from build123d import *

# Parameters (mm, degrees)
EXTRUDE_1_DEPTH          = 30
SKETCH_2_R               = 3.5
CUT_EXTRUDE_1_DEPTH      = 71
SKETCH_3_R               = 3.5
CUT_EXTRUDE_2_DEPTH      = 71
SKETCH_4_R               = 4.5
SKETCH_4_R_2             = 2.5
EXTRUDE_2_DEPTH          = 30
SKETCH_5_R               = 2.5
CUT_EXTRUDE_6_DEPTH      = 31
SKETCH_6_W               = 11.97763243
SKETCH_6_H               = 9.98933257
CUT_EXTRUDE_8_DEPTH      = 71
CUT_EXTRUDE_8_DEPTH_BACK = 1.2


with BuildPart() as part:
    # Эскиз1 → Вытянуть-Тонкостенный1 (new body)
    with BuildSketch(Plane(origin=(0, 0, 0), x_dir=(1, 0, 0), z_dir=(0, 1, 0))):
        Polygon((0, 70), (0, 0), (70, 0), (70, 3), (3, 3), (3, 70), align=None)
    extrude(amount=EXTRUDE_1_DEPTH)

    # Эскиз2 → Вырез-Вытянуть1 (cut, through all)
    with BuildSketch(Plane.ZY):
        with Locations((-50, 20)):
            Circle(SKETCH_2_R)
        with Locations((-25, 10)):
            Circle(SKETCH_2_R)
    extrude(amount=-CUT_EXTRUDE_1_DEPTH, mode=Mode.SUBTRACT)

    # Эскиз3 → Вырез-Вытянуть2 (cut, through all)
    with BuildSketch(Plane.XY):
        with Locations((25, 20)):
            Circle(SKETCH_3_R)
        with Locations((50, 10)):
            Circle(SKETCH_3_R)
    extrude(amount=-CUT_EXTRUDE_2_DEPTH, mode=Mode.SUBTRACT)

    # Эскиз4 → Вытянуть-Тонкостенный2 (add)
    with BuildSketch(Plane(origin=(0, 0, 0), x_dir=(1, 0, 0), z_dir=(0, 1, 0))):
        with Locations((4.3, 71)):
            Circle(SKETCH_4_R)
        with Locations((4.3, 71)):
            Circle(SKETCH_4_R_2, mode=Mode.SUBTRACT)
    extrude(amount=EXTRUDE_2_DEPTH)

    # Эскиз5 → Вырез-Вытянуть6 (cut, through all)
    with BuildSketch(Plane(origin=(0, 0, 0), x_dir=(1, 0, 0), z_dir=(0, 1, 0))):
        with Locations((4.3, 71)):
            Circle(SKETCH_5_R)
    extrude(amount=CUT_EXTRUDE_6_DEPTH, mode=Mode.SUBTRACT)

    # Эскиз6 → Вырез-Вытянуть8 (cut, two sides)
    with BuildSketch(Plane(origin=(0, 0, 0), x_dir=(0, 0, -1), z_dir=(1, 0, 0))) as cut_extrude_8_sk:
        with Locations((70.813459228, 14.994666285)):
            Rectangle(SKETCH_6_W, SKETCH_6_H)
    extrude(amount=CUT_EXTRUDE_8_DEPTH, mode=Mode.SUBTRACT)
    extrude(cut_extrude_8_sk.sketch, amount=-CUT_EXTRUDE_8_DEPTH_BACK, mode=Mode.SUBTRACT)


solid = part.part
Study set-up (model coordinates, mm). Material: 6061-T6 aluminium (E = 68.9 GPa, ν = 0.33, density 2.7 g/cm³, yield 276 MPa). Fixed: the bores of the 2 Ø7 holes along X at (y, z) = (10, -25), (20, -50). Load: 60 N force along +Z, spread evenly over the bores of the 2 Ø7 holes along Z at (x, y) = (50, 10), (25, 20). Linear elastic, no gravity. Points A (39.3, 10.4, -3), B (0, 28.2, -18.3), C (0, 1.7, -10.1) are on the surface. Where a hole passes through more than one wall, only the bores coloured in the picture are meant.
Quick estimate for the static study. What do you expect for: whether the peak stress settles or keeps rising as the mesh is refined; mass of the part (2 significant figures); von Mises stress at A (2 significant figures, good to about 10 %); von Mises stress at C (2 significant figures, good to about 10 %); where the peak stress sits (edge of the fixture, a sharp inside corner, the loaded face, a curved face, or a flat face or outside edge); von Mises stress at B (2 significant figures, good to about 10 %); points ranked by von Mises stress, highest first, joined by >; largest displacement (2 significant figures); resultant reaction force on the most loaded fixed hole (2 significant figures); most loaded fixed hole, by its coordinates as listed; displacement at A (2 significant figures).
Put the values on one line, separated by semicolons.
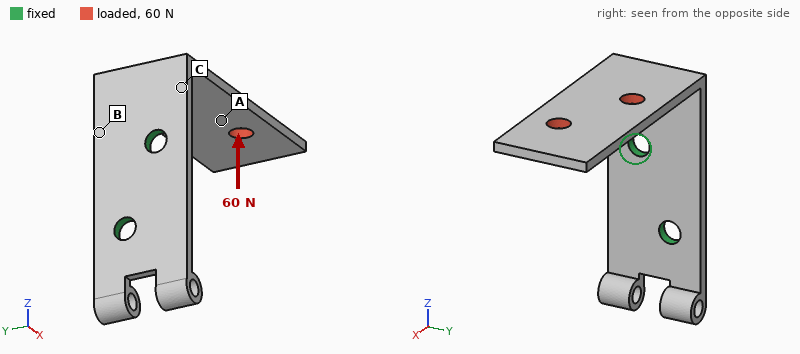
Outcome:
keeps rising; 34 g; 8.6 MPa; 51 MPa; edge of the fixture; 37 MPa; C > B > A; 1.2 mm; 51 N; (10, -25); 0.58 mm
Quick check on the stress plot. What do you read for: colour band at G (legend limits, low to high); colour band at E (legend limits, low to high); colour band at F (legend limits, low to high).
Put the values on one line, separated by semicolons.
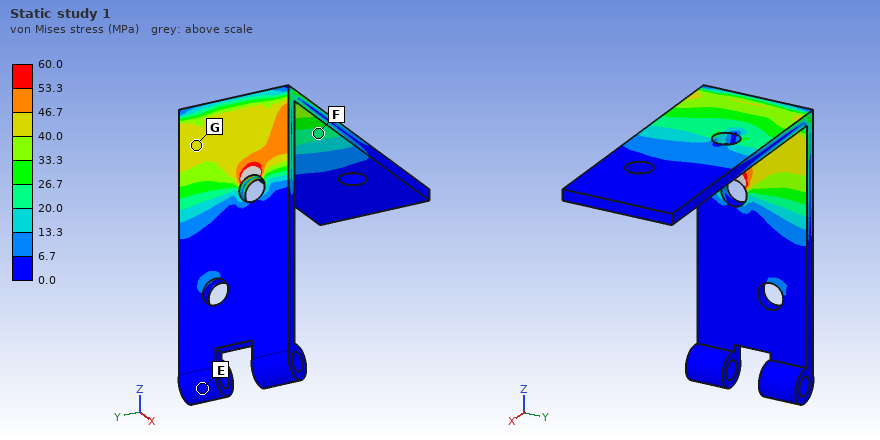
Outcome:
40.0 to 46.7 MPa; 0.0 to 6.7 MPa; 20.0 to 26.7 MPa
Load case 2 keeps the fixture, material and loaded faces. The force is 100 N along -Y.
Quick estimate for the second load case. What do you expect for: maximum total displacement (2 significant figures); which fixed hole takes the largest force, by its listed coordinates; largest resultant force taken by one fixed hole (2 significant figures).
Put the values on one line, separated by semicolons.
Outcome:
0.69 mm; (10, -25); 150 N
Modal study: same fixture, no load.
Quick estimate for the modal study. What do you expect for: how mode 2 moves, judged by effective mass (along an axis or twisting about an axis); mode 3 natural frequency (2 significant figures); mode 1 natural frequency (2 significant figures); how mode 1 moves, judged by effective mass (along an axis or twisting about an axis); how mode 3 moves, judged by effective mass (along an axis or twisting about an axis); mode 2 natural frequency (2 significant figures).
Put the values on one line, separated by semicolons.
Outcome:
along Y; 1700 Hz; 350 Hz; along Z; along X; 600 Hz
